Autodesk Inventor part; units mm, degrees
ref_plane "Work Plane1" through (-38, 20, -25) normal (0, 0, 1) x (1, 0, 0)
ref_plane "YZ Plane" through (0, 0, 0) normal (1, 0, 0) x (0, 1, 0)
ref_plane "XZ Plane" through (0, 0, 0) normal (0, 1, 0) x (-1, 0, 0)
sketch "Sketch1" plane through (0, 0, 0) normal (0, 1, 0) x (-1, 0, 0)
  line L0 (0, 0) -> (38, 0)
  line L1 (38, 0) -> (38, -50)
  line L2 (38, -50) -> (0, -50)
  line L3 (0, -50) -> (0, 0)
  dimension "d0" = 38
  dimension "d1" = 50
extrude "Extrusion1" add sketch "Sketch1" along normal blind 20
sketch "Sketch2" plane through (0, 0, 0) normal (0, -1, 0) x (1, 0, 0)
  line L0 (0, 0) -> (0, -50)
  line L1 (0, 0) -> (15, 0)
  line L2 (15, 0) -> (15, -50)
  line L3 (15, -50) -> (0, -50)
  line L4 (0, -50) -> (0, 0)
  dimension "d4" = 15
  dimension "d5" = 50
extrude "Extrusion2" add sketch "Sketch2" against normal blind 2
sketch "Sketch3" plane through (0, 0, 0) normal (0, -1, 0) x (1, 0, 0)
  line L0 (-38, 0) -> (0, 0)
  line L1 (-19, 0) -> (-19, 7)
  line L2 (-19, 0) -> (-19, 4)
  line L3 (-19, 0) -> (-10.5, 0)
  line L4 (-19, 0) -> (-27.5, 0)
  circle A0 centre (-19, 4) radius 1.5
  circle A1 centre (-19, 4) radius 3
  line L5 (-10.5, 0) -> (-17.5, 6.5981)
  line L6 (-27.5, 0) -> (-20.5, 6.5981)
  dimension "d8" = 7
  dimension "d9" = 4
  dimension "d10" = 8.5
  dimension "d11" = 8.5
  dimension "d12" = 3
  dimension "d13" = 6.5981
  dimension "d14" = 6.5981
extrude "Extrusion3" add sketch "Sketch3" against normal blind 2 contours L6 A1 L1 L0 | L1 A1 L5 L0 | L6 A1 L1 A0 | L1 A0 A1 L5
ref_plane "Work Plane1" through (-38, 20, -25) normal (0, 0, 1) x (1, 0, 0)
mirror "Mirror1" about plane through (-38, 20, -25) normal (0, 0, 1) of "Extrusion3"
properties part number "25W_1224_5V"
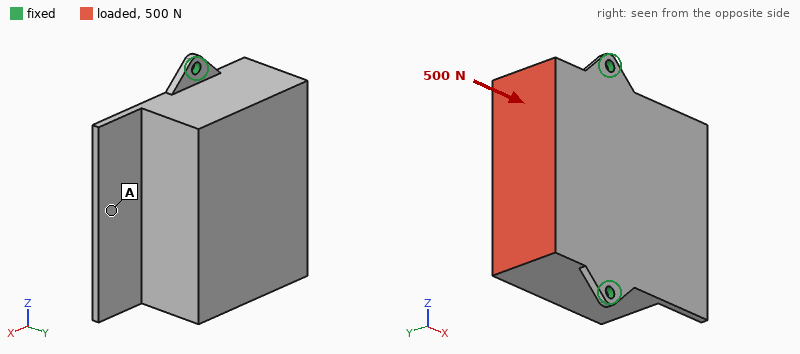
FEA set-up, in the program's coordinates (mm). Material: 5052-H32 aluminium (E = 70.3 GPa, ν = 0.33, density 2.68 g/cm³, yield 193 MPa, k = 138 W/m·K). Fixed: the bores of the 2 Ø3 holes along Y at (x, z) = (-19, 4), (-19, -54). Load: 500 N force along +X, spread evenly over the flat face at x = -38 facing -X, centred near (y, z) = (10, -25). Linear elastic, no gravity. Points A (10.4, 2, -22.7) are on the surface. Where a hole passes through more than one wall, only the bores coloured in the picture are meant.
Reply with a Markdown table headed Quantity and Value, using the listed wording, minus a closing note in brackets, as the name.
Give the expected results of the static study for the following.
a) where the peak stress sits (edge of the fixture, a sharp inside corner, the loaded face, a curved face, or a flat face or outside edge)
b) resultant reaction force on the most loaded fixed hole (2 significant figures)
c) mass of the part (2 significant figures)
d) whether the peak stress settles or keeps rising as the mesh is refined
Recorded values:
| Quantity | Value |
|---|---|
| where the peak stress sits | edge of the fixture |
| resultant reaction force on the most loaded fixed hole | 250 N |
| mass of the part | 110 g |
| whether the peak stress settles or keeps rising as the mesh is refined | keeps rising |
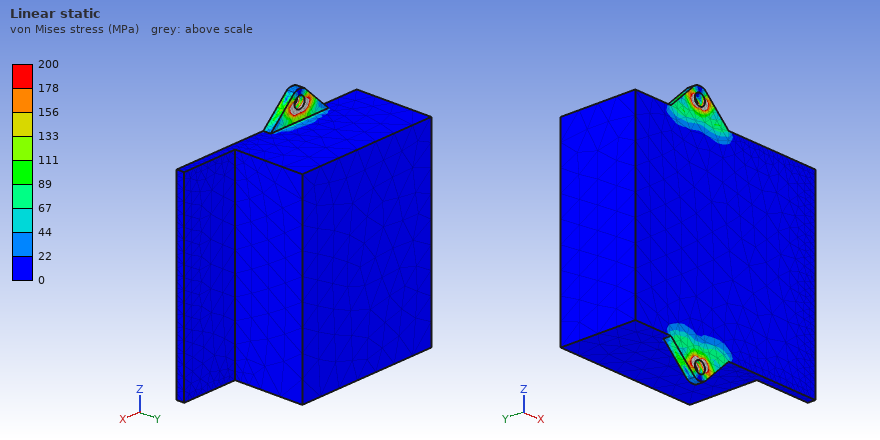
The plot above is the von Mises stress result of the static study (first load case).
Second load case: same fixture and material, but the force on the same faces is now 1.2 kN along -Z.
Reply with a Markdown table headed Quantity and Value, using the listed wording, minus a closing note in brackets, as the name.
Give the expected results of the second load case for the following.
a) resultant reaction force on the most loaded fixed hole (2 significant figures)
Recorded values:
| Quantity | Value |
|---|---|
| resultant reaction force on the most loaded fixed hole | 750 N |
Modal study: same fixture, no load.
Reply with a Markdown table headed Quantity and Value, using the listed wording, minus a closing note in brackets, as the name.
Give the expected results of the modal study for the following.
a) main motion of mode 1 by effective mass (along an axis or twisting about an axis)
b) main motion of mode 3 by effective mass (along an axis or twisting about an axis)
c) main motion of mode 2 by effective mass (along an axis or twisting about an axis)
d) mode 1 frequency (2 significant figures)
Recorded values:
| Quantity | Value |
|---|---|
| main motion of mode 1 by effective mass | along X |
| main motion of mode 3 by effective mass | along Z |
| main motion of mode 2 by effective mass | along Y |
| mode 1 frequency | 730 Hz |
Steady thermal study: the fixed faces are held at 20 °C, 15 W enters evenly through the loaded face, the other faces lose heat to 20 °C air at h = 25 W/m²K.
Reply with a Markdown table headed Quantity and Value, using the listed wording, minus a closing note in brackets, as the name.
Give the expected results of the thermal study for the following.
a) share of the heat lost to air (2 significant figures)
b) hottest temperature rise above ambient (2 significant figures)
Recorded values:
| Quantity | Value |
|---|---|
| share of the heat lost to air | 17 % |
| hottest temperature rise above ambient | 15 K |
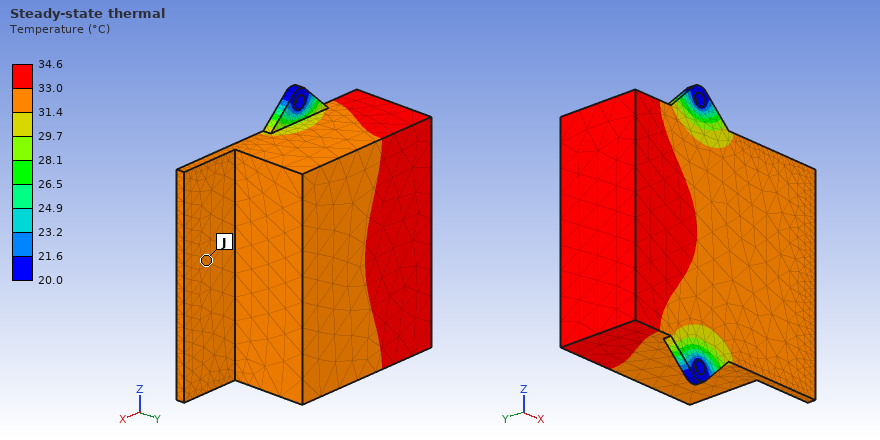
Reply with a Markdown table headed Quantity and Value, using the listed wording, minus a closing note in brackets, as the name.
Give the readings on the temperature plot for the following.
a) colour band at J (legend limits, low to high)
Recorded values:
| Quantity | Value |
|---|---|
| colour band at J | 31.4 to 33.0 °C |
